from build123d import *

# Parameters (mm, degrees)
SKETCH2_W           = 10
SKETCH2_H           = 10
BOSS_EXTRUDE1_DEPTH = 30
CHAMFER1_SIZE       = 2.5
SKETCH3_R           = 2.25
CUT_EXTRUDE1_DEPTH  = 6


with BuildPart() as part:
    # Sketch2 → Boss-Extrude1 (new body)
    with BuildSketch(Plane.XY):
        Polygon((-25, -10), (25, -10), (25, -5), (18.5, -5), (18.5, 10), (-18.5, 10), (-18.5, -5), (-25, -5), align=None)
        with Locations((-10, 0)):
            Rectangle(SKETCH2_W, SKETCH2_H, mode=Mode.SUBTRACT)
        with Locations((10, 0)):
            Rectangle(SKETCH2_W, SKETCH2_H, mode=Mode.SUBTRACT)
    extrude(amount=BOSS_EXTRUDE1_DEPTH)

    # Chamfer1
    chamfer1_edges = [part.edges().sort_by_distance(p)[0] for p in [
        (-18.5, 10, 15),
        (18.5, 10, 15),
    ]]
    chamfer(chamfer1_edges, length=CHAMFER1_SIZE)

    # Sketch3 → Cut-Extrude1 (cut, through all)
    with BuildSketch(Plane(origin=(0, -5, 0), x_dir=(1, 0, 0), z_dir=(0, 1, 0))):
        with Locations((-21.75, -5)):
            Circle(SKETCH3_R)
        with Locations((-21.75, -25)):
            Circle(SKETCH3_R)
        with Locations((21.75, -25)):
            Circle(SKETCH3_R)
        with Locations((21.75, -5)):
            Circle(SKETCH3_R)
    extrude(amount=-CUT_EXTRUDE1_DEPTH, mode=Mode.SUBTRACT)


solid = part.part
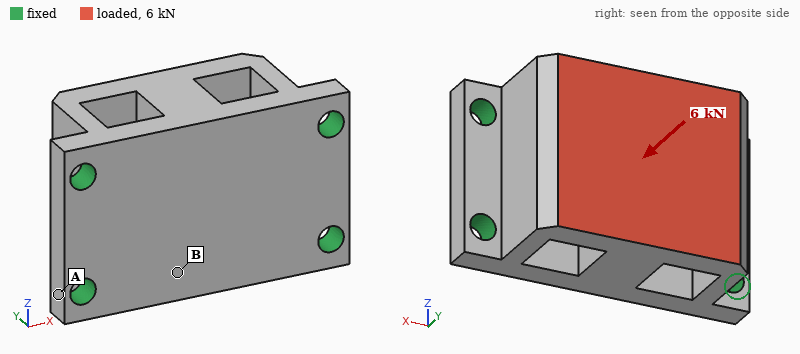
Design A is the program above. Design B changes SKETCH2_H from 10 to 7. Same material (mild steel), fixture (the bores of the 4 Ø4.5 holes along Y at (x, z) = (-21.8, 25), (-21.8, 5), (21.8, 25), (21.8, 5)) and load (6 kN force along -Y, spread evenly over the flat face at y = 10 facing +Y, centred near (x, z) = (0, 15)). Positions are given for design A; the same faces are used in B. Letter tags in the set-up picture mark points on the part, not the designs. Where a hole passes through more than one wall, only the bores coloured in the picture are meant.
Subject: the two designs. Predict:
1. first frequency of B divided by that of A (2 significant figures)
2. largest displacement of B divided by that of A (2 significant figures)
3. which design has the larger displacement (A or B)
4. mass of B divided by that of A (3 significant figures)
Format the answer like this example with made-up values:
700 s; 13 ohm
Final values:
1.0; 0.71; A; 1.10
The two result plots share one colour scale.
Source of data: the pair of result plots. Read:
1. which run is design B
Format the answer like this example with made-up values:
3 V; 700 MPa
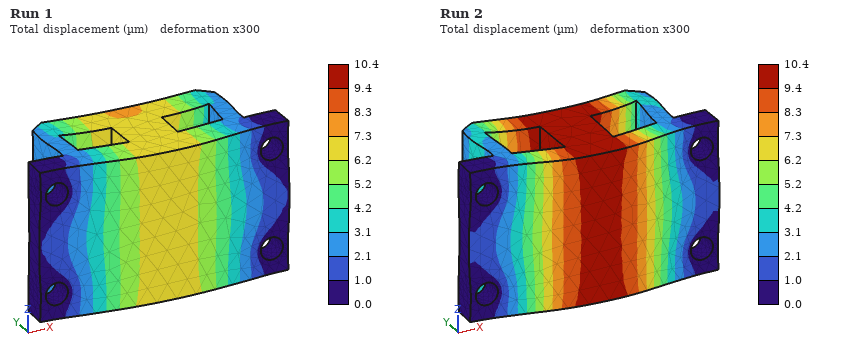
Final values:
Run 1
